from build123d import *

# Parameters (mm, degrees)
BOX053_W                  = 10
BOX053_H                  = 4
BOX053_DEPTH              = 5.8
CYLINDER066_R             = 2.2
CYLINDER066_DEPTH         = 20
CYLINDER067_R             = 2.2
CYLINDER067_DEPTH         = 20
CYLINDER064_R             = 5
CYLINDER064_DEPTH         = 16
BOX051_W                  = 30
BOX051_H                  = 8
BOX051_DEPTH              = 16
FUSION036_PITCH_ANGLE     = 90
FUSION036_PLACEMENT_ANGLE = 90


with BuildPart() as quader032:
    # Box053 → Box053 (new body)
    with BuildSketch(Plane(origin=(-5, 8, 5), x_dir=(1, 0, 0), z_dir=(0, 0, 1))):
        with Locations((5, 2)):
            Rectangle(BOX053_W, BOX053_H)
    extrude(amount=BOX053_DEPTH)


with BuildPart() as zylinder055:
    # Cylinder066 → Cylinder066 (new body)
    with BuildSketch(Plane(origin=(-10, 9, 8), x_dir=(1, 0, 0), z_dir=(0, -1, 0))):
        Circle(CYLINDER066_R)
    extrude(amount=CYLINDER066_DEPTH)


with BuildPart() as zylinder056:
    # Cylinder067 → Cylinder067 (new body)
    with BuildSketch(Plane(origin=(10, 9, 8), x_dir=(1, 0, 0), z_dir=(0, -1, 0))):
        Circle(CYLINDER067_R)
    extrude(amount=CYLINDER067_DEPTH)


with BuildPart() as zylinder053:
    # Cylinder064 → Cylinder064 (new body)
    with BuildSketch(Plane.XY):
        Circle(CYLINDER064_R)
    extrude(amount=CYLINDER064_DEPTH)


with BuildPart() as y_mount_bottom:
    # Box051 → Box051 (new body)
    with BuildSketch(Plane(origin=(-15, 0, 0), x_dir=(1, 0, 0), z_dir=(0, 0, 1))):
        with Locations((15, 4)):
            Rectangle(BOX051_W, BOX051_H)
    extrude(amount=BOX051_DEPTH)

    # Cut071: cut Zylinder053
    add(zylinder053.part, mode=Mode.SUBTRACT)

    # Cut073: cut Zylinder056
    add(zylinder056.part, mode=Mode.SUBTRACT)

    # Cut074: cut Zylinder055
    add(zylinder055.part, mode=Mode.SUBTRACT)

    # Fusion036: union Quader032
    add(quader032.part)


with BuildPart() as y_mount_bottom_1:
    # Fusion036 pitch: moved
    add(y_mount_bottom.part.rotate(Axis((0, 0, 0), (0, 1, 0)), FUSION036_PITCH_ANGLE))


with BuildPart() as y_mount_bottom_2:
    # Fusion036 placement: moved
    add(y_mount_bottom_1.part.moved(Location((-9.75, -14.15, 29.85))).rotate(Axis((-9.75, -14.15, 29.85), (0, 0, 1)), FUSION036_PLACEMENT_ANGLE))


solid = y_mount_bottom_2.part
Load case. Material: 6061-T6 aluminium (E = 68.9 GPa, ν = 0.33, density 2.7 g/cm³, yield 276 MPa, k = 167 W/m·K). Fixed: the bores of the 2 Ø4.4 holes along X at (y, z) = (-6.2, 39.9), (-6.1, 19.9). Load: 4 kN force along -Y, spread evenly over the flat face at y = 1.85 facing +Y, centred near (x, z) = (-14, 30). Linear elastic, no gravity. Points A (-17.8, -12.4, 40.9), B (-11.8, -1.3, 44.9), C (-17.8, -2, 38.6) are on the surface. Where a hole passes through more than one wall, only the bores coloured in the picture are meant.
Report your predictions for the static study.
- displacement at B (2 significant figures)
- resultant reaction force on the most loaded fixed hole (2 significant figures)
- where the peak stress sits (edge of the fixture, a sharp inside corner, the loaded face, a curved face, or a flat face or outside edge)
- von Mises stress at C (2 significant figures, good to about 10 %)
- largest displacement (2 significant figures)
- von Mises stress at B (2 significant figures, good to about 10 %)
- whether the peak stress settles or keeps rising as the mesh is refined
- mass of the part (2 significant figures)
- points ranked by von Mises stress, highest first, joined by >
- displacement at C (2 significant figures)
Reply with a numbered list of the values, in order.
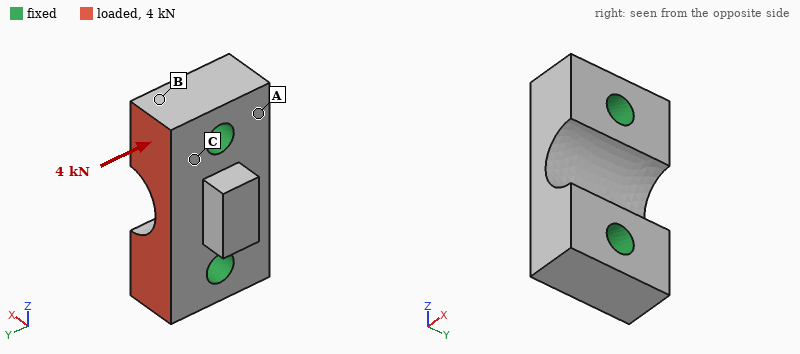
1. 1.4 µm
2. 2.0 kN
3. edge of the fixture
4. 28 MPa
5. 4.6 µm
6. 16 MPa
7. keeps rising
8. 8.6 g
9. C > B > A
10. 1.2 µm
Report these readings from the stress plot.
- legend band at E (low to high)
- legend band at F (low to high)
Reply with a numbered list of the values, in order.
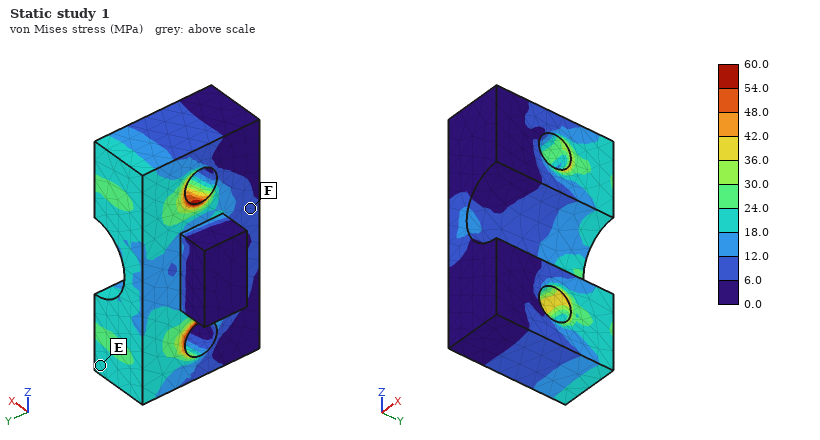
1. 18.0 to 24.0 MPa
2. 6.0 to 12.0 MPa
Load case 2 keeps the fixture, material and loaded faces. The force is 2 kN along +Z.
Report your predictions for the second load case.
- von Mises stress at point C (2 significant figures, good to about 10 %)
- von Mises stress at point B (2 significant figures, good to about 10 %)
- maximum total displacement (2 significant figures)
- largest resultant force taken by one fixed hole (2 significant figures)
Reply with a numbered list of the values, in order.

1. 26 MPa
2. 18 MPa
3. 6.6 µm
4. 1.1 kN
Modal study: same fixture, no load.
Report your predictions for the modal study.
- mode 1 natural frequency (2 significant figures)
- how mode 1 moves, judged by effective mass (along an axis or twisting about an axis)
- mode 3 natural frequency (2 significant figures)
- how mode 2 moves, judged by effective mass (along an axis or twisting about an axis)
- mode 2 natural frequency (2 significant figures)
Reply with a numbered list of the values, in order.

1. 49 kHz
2. along Y
3. 71 kHz
4. along X
5. 62 kHz
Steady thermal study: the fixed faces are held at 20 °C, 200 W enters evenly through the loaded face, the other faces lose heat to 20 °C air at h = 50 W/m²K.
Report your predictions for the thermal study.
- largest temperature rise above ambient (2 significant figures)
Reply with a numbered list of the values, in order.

1. 49 K
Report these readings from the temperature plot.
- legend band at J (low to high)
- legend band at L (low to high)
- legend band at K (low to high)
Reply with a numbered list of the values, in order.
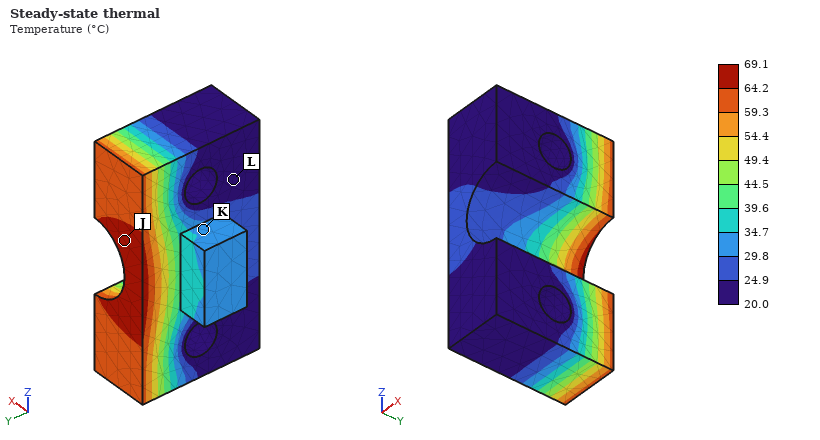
1. 64.2 to 69.1 °C
2. 20.0 to 24.9 °C
3. 29.8 to 34.7 °C
